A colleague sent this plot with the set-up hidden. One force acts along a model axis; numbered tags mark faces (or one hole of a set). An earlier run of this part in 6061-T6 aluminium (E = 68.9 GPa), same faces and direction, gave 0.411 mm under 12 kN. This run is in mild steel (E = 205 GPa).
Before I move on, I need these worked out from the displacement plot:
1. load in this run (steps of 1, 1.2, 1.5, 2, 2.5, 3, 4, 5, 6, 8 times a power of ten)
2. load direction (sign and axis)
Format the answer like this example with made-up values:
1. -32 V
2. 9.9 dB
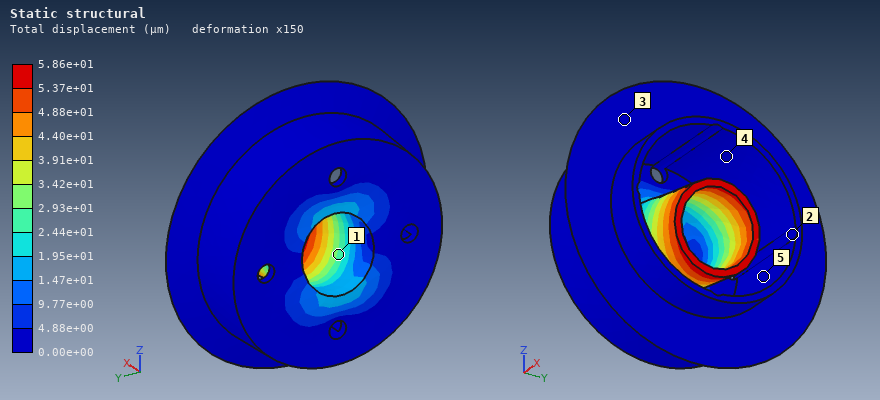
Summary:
1. 5 kN
2. -Z
